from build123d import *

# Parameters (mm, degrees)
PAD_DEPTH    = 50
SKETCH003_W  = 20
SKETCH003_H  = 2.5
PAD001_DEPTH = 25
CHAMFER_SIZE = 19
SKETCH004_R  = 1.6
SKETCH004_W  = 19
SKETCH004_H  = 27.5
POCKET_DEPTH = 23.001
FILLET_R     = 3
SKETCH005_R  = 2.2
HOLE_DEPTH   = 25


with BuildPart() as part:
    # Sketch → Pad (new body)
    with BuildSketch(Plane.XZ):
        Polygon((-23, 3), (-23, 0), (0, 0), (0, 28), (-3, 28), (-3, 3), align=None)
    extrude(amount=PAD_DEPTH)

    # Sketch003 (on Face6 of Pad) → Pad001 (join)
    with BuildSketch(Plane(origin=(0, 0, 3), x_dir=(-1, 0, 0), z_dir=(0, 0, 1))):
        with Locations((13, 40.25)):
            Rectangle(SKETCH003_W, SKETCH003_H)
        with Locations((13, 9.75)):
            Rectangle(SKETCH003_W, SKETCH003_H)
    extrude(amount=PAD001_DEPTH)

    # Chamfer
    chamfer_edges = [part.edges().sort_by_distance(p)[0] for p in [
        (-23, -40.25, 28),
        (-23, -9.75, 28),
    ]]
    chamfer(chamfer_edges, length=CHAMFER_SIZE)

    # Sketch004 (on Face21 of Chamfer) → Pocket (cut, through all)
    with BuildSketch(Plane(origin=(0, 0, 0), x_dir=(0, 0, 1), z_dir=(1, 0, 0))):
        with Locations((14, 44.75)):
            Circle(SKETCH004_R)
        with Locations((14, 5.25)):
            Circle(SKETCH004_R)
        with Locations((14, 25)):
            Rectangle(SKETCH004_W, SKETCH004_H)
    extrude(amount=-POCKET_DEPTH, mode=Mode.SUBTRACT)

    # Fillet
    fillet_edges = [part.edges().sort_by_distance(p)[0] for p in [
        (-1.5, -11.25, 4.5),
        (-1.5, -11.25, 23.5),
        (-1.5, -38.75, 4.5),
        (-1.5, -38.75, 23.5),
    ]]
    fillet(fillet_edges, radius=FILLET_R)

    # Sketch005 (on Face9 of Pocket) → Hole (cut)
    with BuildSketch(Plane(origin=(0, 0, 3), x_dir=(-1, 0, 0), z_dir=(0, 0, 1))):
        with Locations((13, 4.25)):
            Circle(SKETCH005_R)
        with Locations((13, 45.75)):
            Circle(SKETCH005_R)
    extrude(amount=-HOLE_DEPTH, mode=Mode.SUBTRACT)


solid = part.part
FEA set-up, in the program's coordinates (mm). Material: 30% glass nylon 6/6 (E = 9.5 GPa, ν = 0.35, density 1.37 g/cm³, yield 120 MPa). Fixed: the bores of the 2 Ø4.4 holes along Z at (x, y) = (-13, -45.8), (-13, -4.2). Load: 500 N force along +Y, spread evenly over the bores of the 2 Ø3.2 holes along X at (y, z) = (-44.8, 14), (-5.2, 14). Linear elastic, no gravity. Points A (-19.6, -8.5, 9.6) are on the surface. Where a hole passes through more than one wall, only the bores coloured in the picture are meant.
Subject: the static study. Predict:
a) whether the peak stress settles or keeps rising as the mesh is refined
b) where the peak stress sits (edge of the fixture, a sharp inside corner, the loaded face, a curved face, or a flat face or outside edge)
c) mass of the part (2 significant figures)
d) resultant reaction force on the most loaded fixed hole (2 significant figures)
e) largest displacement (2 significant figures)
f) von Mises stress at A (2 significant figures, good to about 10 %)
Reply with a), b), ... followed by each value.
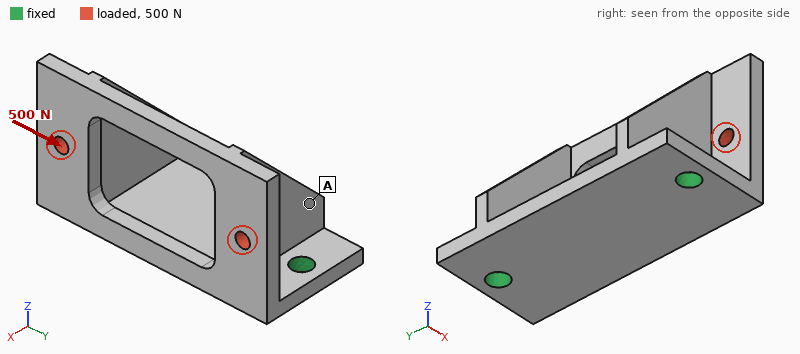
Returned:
a) keeps rising
b) edge of the fixture
c) 9.7 g
d) 310 N
e) 0.42 mm
f) 12 MPa
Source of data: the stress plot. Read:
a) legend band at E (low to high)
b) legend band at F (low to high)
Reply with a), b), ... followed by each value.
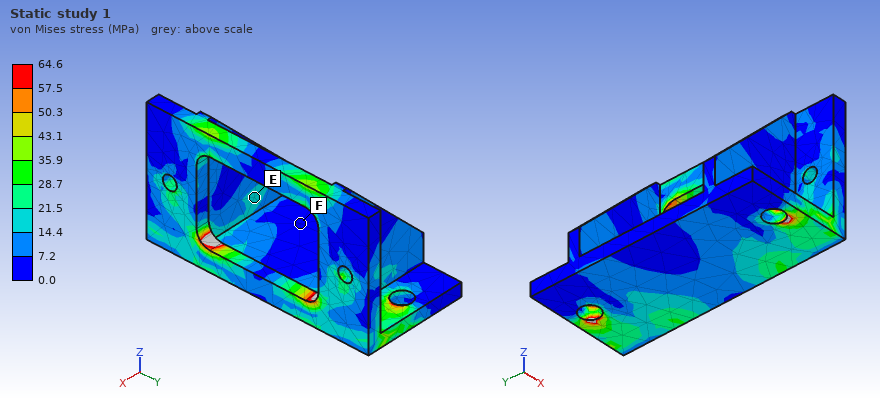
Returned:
a) 14.4 to 21.5 MPa
b) 0.0 to 7.2 MPa
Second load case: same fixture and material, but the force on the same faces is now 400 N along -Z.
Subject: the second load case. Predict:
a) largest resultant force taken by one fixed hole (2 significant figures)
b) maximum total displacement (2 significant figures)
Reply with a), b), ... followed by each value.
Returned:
a) 200 N
b) 0.37 mm
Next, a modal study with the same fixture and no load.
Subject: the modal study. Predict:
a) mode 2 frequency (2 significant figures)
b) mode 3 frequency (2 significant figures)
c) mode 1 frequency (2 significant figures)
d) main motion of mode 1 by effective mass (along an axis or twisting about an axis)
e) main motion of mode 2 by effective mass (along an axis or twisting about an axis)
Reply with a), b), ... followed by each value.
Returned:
a) 2700 Hz
b) 3300 Hz
c) 2200 Hz
d) along X
e) along Y
